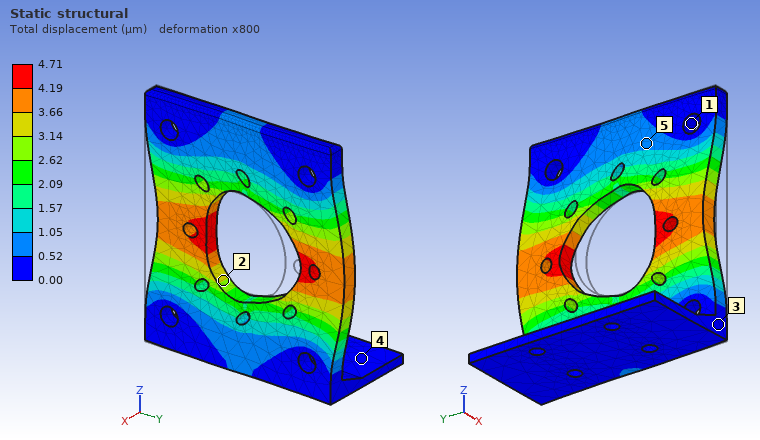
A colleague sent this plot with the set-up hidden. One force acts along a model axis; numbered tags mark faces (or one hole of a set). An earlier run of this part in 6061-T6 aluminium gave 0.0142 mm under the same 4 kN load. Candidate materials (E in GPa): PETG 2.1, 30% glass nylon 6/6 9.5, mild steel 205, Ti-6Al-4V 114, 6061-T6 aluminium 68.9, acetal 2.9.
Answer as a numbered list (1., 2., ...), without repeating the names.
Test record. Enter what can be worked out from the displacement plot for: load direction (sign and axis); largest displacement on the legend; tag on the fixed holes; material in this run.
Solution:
1. +Y
2. 4.71 µm
3. 1
4. mild steel
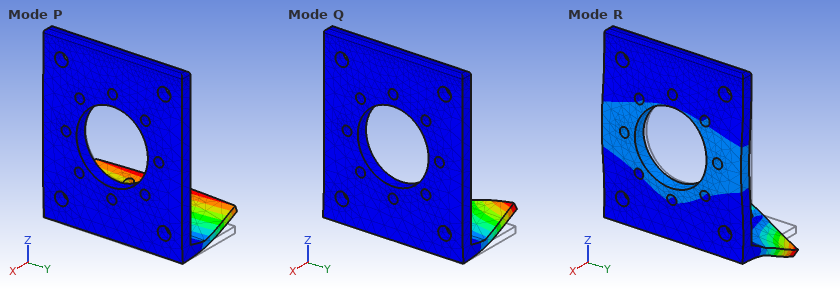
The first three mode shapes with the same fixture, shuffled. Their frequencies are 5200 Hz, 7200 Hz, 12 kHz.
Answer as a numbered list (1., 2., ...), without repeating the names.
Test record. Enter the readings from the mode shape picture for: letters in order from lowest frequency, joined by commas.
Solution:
1. P, Q, R
